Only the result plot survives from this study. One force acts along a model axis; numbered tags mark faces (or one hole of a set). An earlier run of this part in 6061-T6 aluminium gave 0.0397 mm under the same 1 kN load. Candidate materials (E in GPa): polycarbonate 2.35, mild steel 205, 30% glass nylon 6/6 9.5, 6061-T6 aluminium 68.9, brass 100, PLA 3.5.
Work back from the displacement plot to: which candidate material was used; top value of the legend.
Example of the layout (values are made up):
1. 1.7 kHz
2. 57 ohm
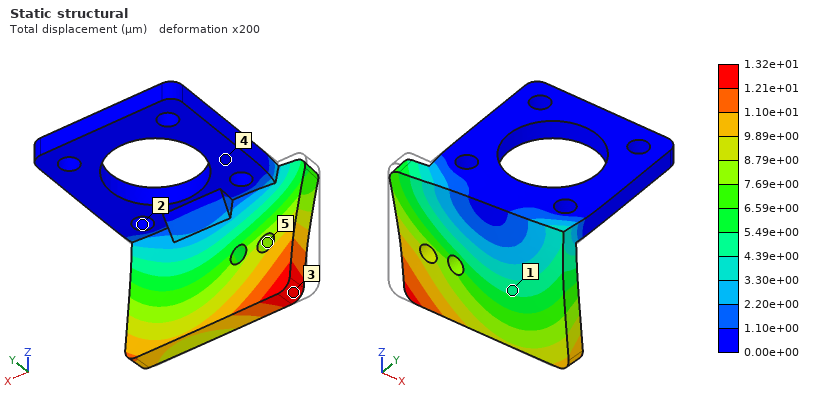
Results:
1. mild steel
2. 1.32e+01 µm
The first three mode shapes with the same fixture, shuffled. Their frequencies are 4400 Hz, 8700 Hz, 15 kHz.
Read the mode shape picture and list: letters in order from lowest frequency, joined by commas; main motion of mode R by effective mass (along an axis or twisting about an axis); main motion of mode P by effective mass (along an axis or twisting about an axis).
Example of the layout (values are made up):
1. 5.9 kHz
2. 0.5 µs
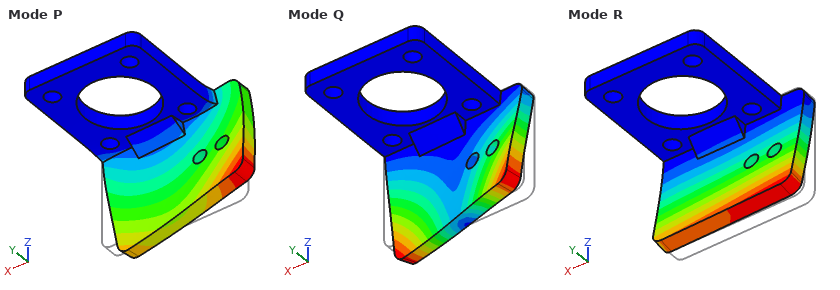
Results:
1. R, Q, P
2. along Y
3. along X
